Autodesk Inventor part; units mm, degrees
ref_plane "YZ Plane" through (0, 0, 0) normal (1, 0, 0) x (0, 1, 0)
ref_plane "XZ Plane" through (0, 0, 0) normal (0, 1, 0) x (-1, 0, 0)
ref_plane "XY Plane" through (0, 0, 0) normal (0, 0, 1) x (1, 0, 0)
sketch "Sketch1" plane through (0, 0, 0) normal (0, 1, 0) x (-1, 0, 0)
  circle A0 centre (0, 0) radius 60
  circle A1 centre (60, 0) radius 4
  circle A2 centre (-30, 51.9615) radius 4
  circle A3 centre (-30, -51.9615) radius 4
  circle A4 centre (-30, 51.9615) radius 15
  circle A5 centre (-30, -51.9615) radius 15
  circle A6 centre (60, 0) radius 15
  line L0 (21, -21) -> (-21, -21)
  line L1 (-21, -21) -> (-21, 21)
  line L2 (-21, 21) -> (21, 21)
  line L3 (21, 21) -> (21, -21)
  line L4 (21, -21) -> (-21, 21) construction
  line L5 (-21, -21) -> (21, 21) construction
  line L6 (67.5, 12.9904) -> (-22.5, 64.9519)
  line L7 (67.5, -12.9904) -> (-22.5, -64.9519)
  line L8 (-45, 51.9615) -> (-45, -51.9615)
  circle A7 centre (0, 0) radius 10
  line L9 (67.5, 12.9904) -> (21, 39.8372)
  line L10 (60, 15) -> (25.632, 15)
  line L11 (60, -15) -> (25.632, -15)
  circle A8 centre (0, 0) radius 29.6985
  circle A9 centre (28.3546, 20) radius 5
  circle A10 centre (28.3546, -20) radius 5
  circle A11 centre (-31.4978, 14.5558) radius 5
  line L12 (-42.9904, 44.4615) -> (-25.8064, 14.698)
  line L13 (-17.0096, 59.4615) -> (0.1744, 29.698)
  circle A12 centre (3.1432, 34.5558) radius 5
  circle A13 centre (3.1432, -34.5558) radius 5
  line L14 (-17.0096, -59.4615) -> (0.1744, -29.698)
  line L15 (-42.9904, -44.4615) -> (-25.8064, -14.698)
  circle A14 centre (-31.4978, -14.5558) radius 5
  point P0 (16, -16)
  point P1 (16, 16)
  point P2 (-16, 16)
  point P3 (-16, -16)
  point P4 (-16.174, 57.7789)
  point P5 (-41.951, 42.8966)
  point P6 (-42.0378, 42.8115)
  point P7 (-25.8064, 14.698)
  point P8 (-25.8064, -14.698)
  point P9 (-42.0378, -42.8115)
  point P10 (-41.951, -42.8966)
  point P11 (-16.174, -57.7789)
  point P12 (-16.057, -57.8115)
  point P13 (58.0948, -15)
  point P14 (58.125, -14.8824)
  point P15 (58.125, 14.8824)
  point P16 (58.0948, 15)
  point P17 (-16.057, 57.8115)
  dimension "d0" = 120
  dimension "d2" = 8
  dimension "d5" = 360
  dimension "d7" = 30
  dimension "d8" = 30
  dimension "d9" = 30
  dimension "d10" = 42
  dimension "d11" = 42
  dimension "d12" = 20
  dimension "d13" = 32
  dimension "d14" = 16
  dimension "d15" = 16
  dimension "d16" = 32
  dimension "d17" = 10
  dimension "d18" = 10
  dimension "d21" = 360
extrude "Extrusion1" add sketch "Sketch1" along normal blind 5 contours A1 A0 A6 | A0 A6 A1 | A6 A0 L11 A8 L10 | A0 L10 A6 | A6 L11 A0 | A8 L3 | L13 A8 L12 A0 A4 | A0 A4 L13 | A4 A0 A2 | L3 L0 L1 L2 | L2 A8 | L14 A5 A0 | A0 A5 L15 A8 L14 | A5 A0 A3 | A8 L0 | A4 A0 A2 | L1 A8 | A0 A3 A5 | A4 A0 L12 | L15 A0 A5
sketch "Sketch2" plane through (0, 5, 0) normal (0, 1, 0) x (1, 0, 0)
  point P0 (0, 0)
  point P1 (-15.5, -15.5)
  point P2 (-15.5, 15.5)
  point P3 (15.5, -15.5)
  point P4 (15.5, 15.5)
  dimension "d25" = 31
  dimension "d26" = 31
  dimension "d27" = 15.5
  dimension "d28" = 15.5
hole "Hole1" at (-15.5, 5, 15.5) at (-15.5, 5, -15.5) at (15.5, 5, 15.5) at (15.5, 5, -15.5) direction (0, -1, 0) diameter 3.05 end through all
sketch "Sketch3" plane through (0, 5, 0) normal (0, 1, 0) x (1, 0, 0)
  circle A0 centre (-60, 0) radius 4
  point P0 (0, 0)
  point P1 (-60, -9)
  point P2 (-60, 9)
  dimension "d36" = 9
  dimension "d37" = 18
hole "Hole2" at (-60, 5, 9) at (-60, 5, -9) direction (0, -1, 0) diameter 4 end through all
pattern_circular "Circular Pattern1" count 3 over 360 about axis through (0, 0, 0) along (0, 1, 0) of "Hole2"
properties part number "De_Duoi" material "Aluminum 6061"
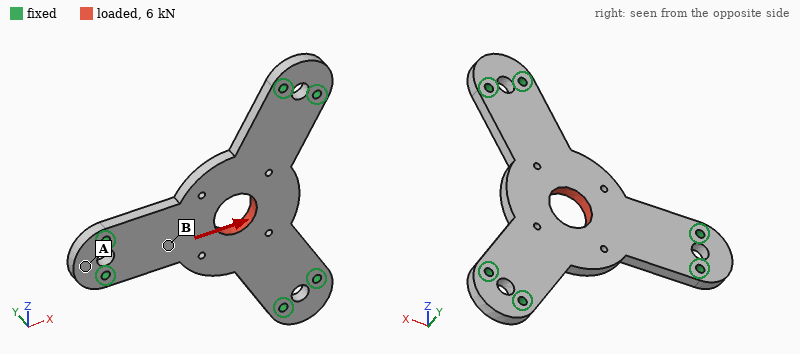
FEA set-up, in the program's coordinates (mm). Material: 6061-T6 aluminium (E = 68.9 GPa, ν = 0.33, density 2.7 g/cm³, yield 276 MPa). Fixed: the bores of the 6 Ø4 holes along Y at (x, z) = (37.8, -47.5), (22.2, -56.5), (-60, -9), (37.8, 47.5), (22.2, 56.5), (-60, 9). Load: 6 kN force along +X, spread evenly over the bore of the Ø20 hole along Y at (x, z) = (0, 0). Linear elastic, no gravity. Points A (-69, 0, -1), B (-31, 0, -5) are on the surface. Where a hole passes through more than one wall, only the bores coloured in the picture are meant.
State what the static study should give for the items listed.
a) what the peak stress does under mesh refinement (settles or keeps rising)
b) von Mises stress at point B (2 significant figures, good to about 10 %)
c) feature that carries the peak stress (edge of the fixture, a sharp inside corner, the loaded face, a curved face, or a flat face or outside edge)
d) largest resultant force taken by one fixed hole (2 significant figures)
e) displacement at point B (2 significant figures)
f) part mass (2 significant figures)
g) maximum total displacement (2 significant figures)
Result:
keeps rising
19 MPa
edge of the fixture
1.8 kN
9.7 µm
82 g
30 µm
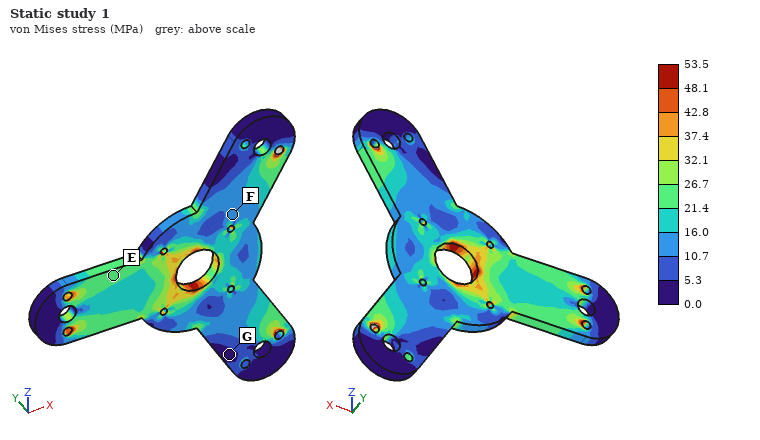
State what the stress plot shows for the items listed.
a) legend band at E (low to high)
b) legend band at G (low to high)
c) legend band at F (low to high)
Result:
21.4 to 26.7 MPa
0.0 to 5.3 MPa
10.7 to 16.0 MPa
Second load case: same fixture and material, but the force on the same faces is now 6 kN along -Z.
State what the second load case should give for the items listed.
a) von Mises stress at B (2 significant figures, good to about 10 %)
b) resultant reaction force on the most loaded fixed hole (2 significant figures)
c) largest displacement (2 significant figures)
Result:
10 MPa
2.0 kN
29 µm
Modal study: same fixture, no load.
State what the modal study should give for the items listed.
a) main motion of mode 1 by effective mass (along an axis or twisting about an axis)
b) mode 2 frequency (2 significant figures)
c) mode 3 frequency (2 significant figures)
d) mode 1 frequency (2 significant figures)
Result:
along Y
4300 Hz
4300 Hz
2100 Hz
